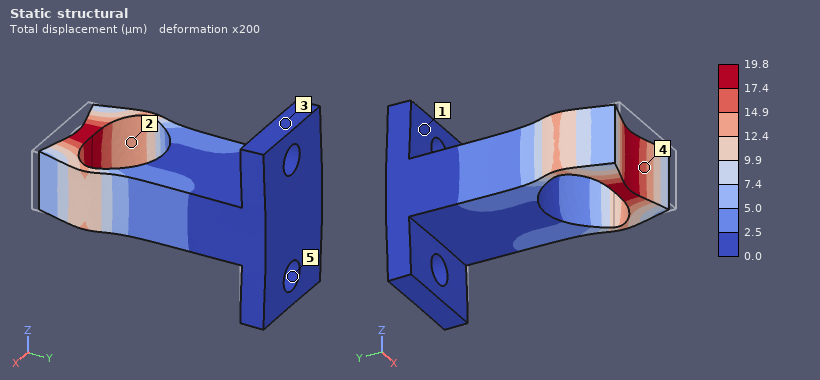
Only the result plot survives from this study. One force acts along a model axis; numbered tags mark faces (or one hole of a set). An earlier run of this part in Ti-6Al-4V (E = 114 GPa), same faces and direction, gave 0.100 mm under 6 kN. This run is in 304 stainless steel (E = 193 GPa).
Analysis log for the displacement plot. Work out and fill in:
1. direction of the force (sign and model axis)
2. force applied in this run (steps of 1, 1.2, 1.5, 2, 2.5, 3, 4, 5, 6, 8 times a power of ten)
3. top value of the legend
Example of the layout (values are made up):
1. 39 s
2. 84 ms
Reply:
1. +Y
2. 2 kN
3. 19.8 µm
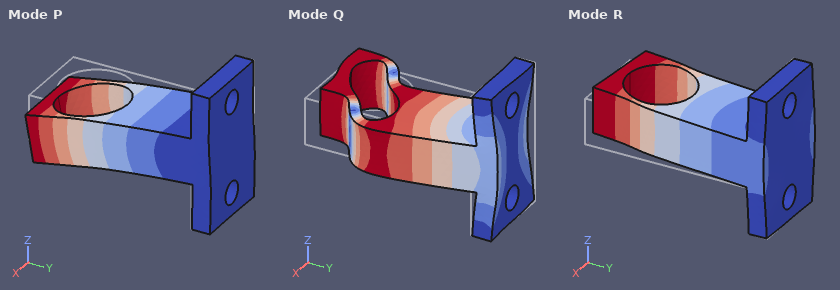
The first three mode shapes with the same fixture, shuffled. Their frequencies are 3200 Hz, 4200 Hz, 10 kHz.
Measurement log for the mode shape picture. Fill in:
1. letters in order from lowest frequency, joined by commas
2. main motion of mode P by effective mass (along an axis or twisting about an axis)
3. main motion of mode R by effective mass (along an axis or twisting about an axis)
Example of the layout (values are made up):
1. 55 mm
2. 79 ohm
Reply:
1. R, P, Q
2. along Z
3. along X
